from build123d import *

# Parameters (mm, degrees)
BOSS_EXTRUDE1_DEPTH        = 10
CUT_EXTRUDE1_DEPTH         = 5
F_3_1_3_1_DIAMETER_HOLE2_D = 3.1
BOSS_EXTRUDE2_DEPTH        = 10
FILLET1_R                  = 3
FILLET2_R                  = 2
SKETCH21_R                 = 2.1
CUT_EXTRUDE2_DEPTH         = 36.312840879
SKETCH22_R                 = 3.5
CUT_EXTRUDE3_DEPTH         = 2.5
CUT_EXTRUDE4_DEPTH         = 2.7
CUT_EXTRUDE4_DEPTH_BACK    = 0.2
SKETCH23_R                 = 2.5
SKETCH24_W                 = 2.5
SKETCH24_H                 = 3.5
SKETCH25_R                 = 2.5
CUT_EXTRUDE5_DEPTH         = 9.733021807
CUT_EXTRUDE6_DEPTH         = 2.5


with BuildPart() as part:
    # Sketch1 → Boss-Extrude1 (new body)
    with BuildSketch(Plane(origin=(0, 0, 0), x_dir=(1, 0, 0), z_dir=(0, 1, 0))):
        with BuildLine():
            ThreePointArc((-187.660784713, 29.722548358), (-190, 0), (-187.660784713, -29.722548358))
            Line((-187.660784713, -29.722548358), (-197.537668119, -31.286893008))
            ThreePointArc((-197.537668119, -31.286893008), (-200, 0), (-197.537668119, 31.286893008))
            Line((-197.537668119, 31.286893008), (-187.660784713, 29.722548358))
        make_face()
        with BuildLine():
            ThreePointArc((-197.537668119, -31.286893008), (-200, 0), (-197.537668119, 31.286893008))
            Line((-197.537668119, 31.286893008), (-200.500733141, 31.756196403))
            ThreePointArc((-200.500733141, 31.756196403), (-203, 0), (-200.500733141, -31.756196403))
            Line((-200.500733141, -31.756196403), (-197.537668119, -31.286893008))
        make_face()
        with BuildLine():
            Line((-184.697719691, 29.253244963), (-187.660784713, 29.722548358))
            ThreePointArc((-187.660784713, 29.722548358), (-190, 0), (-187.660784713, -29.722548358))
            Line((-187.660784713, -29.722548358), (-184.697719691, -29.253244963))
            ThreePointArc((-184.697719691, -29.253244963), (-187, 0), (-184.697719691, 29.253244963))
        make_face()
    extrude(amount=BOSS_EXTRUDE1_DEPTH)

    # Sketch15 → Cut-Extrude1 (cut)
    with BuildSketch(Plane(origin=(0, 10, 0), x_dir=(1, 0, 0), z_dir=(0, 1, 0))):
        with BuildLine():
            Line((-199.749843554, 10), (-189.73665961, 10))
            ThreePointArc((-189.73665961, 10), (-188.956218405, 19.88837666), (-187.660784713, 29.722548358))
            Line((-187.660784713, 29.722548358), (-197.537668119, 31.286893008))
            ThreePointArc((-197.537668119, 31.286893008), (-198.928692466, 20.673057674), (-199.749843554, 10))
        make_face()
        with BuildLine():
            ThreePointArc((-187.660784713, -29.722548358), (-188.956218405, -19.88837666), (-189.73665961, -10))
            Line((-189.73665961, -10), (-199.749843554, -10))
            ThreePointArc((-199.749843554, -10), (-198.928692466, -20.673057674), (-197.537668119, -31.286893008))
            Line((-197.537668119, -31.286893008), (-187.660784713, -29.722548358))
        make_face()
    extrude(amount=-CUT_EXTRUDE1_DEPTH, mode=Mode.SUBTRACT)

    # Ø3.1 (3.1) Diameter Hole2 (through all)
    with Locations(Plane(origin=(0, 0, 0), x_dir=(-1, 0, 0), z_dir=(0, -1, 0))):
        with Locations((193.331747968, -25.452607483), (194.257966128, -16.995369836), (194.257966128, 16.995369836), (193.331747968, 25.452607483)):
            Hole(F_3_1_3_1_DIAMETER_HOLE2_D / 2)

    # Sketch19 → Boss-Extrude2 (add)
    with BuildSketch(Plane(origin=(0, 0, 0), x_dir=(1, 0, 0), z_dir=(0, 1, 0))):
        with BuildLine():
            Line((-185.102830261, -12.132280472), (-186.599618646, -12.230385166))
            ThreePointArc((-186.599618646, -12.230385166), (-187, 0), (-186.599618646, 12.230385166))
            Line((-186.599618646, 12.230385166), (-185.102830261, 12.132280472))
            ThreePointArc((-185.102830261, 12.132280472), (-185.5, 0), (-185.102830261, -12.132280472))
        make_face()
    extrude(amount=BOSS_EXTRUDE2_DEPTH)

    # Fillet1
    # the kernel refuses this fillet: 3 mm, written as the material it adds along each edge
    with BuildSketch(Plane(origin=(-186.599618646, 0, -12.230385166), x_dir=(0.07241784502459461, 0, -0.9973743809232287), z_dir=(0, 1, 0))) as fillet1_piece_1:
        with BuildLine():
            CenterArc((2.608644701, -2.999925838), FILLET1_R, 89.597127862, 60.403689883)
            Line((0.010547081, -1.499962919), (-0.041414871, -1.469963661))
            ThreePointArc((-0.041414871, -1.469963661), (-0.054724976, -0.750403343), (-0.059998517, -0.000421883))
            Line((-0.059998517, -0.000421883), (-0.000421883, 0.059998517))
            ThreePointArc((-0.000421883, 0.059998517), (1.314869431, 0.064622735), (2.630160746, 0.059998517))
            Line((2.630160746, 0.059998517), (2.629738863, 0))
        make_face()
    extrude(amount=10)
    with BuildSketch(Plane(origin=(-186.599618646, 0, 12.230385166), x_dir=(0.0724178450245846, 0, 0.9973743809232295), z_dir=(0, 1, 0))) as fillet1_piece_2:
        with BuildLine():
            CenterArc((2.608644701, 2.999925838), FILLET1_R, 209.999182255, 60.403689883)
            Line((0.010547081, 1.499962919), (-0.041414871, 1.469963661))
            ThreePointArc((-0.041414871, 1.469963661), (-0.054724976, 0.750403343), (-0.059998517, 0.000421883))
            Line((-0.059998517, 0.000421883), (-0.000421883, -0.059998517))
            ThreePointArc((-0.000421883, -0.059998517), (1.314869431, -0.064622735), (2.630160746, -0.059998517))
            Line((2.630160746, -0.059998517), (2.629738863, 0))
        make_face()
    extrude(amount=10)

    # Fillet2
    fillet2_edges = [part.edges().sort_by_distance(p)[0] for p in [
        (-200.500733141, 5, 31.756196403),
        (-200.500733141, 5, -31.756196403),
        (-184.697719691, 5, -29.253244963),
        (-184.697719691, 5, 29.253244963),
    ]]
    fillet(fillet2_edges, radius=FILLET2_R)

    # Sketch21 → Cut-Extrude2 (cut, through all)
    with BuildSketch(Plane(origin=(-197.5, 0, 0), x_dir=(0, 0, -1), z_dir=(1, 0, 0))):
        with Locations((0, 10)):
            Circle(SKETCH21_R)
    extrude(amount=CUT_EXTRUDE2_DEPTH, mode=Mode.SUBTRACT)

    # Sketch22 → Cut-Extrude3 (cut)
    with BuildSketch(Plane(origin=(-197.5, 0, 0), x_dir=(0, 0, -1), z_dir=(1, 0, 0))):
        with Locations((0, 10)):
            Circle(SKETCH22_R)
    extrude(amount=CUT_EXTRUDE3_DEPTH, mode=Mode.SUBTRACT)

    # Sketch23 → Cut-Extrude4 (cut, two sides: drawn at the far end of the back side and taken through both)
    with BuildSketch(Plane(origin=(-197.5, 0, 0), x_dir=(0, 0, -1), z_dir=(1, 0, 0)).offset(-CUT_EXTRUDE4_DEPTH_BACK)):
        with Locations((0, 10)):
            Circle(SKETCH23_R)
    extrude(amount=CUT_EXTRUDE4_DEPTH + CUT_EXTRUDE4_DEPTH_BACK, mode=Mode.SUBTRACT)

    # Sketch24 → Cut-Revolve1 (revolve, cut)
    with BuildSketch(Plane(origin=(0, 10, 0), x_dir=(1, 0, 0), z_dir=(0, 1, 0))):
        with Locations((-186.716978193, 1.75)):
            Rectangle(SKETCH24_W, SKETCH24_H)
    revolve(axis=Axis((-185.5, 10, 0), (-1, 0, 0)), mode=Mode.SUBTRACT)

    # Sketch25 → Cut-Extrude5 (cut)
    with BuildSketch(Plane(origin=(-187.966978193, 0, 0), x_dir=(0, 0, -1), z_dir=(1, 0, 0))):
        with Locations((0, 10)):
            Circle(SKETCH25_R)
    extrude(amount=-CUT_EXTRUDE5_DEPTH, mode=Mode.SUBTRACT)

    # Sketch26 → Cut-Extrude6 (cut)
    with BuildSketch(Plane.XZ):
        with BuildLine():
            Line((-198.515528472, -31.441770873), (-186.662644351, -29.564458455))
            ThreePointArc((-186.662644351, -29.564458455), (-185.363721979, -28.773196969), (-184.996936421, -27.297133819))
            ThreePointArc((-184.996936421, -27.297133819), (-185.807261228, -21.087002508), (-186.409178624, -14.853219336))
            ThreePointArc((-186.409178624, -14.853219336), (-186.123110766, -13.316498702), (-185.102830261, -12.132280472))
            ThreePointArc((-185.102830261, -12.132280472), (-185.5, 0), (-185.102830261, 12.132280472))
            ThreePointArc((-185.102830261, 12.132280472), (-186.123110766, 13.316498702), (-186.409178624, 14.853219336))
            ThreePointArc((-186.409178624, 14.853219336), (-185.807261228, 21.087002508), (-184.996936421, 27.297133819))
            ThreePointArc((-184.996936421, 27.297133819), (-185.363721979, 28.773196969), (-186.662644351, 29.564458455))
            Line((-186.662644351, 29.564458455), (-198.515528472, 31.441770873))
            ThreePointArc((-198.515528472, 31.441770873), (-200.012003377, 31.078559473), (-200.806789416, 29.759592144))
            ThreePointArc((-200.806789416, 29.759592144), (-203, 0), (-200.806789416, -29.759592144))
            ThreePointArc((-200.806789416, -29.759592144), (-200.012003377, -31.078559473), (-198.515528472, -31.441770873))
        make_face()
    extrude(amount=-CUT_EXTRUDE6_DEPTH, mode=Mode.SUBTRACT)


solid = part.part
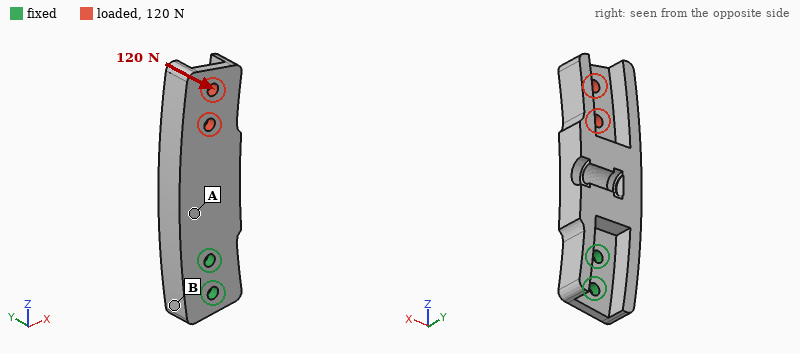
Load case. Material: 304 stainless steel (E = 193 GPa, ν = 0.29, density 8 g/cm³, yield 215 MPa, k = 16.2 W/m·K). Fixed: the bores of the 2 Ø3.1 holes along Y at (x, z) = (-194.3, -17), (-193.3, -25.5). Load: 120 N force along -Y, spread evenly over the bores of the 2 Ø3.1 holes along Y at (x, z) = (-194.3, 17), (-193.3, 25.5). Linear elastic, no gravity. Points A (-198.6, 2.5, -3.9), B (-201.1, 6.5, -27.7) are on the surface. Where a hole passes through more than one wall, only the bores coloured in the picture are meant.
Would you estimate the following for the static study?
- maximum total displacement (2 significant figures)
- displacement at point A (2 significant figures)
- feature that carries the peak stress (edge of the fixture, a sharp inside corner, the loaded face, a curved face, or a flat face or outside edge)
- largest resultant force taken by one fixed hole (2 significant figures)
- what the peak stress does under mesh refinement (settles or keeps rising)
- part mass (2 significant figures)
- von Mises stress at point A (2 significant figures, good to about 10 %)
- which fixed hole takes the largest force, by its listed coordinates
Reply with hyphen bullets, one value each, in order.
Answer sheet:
- 76 µm
- 14 µm
- edge of the fixture
- 490 N
- keeps rising
- 42 g
- 25 MPa
- (-194.3, -17)
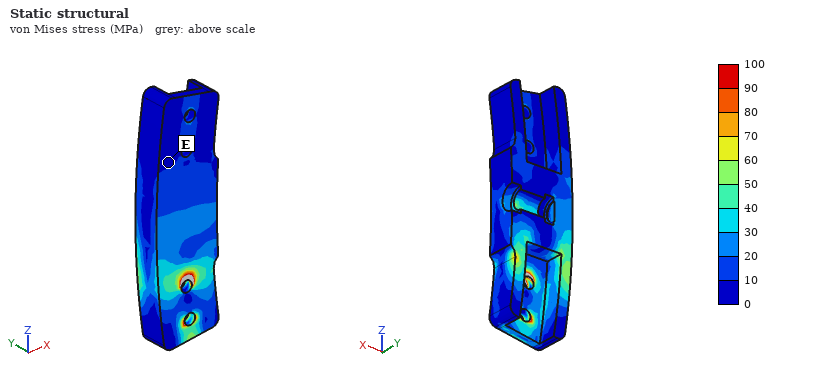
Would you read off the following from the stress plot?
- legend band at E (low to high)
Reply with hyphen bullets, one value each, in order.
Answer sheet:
- 0 to 10 MPa
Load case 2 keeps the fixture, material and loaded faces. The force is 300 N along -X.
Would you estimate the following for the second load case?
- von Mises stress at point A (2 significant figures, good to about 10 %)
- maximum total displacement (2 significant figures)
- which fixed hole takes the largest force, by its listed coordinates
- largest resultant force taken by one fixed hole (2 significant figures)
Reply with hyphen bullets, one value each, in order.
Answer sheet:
- 18 MPa
- 45 µm
- (-194.3, -17)
- 1.2 kN
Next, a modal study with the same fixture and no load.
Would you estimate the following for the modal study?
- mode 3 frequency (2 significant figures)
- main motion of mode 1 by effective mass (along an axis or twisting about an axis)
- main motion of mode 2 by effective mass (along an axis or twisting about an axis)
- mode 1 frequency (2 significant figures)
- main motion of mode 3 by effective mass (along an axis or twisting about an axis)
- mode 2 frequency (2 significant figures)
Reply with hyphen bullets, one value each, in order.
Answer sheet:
- 5800 Hz
- along Y
- along X
- 1900 Hz
- twisting about Z
- 3900 Hz
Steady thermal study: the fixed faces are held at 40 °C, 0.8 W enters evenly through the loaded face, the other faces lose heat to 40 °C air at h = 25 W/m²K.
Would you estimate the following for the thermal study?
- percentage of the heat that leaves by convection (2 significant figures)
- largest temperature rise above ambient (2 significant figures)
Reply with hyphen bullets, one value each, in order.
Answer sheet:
- 62 %
- 15 K
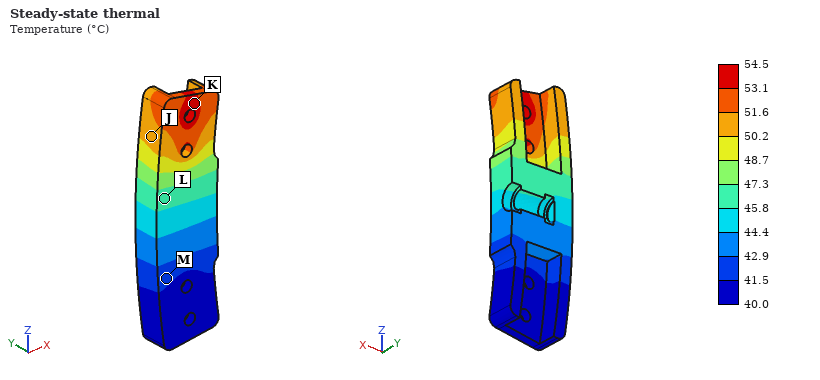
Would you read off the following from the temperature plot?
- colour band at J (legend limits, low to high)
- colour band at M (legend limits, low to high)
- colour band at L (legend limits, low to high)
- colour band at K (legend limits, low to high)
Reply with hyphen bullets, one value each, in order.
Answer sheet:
- 50.2 to 51.6 °C
- 41.5 to 42.9 °C
- 45.8 to 47.3 °C
- 53.1 to 54.5 °C
